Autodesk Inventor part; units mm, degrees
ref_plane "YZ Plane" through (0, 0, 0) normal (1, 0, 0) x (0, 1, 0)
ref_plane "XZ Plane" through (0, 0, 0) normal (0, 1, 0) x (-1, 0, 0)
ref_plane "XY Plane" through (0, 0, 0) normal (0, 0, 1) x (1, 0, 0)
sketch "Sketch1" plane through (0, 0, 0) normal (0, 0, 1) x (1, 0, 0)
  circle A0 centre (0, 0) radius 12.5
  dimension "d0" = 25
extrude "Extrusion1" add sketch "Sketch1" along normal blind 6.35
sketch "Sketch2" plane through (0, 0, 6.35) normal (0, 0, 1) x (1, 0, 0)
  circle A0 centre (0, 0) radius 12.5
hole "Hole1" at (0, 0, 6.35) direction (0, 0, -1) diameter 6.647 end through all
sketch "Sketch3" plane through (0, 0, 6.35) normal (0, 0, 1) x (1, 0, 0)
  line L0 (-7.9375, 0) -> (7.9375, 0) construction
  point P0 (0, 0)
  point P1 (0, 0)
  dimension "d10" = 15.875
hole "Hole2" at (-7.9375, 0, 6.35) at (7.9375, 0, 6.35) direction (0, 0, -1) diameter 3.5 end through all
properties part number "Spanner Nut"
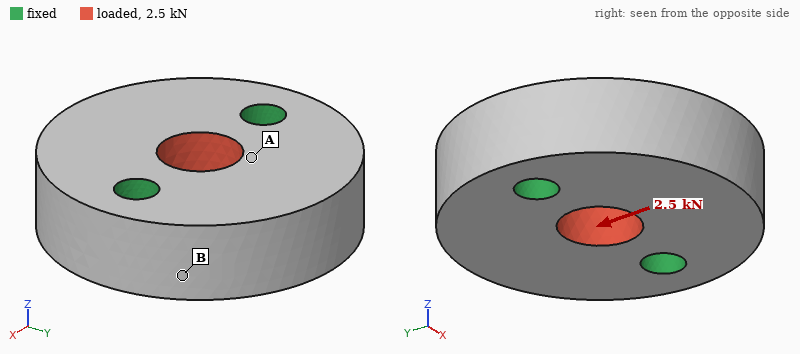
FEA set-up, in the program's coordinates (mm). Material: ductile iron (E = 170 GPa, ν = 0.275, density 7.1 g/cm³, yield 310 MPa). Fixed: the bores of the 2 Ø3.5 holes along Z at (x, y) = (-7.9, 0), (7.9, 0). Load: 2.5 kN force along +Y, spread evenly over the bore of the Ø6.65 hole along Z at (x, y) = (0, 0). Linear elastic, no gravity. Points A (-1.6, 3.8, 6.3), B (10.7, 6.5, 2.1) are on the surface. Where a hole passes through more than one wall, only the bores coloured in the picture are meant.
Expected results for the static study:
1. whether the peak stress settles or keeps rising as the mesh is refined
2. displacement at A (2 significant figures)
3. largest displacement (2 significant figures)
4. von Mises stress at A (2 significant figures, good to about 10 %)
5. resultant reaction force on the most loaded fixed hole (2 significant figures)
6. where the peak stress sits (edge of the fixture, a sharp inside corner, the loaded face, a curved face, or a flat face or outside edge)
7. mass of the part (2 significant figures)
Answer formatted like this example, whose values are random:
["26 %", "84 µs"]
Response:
["keeps rising", "1.1 µm", "1.3 µm", "20 MPa", "1.3 kN", "edge of the fixture", "20 g"]
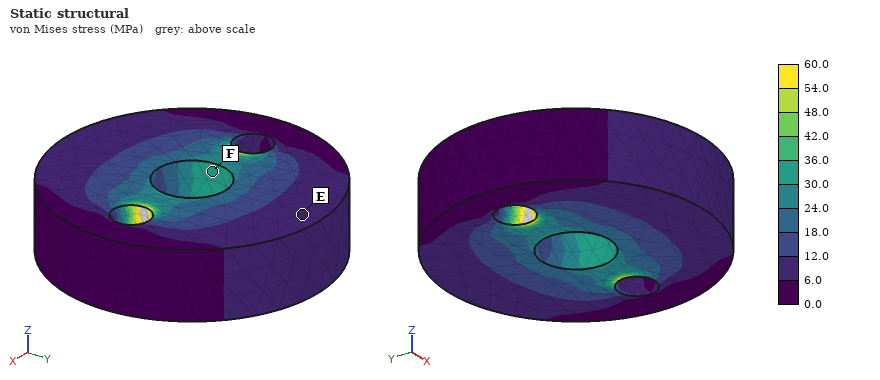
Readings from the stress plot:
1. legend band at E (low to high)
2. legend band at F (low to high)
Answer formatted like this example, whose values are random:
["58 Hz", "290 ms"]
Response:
["6.0 to 12.0 MPa", "30.0 to 36.0 MPa"]
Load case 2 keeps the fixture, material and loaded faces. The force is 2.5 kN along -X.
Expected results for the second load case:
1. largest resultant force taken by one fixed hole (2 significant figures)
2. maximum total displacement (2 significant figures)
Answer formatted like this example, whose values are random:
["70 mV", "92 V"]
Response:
["1.3 kN", "0.98 µm"]
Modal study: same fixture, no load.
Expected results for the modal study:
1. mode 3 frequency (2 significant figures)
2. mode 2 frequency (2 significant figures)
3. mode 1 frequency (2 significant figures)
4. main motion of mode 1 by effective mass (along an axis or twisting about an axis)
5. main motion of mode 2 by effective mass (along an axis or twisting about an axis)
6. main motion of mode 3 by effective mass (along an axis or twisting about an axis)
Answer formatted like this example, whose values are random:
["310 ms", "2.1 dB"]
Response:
["58 kHz", "33 kHz", "30 kHz", "twisting about X", "along Z", "twisting about Z"]
